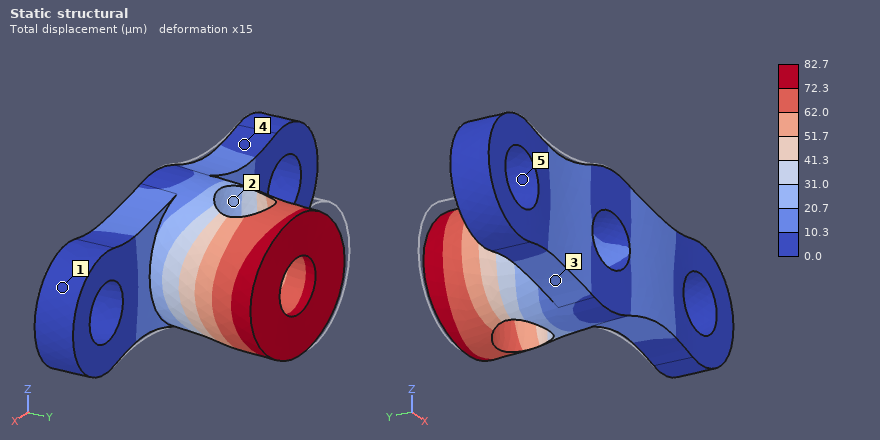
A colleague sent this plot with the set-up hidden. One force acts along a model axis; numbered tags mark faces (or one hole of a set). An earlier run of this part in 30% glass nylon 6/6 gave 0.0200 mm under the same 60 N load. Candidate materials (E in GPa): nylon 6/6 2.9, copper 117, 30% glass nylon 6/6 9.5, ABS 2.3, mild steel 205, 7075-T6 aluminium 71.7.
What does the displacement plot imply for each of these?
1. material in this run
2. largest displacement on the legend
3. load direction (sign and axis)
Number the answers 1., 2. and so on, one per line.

1. ABS
2. 82.7 µm
3. +X
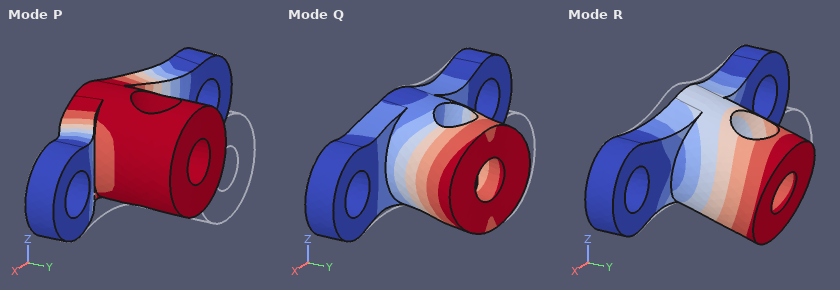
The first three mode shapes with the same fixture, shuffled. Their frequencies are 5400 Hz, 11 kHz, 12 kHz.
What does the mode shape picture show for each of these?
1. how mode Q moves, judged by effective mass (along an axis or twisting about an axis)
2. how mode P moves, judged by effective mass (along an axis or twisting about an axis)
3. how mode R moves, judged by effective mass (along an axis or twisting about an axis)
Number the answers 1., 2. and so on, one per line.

1. along X
2. along Y
3. along Z
